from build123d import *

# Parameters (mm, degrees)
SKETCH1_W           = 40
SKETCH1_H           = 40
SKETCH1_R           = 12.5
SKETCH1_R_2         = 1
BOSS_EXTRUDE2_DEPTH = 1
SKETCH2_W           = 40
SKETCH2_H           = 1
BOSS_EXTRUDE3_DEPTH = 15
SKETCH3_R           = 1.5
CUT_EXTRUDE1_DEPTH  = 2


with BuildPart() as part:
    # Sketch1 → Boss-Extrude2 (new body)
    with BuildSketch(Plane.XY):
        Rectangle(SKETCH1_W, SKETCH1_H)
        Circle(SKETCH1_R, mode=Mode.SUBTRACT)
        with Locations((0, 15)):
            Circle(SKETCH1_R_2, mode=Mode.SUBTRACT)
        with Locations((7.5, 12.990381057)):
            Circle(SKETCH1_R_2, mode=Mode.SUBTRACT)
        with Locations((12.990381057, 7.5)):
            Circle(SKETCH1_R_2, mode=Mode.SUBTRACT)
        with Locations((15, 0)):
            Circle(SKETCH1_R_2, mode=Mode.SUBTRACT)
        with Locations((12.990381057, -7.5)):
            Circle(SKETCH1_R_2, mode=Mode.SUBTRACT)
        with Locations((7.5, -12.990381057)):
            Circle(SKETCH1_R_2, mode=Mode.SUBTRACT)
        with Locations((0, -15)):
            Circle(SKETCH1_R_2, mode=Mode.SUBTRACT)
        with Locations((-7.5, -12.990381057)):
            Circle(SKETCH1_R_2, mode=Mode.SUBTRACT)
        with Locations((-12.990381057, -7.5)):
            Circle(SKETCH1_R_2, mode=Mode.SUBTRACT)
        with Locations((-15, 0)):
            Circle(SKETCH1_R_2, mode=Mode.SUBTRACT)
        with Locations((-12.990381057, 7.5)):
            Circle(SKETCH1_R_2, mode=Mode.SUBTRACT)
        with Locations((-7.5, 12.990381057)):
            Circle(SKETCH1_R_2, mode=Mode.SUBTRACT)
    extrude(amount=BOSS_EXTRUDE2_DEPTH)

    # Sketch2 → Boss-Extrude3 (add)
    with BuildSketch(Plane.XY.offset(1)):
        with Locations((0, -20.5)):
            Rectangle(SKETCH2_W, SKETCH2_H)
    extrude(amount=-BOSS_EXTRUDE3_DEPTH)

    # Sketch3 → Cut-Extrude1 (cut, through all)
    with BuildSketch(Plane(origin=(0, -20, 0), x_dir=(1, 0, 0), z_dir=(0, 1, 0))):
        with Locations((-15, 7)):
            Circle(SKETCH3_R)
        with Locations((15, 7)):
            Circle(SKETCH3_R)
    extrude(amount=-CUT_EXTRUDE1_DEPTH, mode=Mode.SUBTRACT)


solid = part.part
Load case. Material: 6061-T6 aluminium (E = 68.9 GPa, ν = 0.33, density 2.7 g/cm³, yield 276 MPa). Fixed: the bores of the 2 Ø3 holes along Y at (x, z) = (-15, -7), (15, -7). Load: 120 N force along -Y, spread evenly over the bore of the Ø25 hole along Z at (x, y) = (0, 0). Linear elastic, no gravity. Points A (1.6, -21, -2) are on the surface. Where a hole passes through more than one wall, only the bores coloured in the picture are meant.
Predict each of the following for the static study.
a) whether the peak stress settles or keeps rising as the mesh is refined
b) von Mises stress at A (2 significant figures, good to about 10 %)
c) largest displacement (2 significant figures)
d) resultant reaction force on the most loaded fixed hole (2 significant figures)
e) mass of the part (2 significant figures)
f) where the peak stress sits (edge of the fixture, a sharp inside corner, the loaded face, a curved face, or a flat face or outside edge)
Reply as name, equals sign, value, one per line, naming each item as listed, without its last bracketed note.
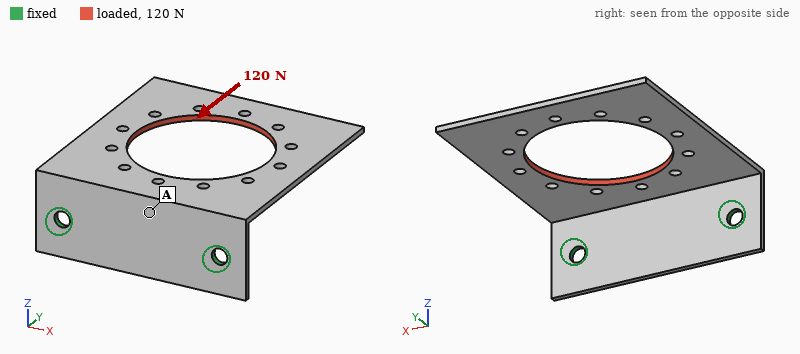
whether the peak stress settles or keeps rising as the mesh is refined = keeps rising
von Mises stress at A = 22 MPa
largest displacement = 0.62 mm
resultant reaction force on the most loaded fixed hole = 60 N
mass of the part = 4.5 g
where the peak stress sits = edge of the fixture
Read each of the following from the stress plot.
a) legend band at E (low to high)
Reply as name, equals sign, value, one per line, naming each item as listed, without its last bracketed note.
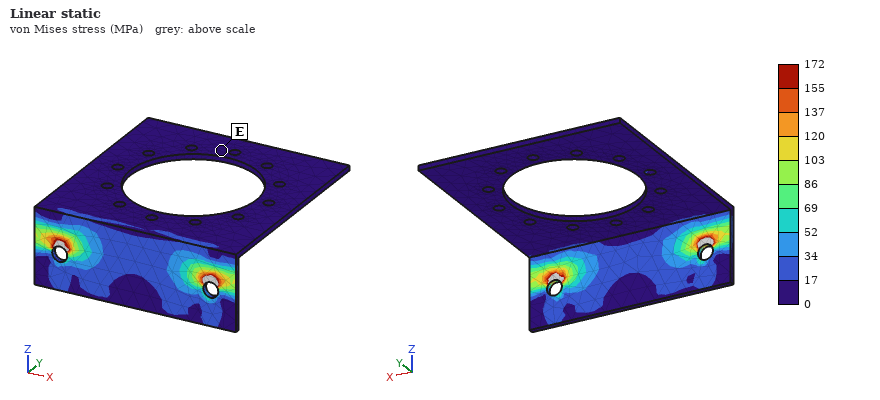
legend band at E = 0 to 17 MPa
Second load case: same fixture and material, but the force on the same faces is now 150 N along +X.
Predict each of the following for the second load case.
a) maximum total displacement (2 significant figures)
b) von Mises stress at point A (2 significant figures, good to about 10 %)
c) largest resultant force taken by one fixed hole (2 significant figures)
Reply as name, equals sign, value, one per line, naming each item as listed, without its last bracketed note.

maximum total displacement = 0.44 mm
von Mises stress at point A = 30 MPa
largest resultant force taken by one fixed hole = 130 N
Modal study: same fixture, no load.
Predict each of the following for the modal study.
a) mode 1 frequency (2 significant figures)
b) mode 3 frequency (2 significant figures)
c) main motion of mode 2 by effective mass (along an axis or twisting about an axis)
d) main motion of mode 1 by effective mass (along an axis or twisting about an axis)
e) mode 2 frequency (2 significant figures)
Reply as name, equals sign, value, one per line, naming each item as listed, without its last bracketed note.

mode 1 frequency = 370 Hz
mode 3 frequency = 2200 Hz
main motion of mode 2 by effective mass = twisting about Y
main motion of mode 1 by effective mass = along Z
mode 2 frequency = 920 Hz
